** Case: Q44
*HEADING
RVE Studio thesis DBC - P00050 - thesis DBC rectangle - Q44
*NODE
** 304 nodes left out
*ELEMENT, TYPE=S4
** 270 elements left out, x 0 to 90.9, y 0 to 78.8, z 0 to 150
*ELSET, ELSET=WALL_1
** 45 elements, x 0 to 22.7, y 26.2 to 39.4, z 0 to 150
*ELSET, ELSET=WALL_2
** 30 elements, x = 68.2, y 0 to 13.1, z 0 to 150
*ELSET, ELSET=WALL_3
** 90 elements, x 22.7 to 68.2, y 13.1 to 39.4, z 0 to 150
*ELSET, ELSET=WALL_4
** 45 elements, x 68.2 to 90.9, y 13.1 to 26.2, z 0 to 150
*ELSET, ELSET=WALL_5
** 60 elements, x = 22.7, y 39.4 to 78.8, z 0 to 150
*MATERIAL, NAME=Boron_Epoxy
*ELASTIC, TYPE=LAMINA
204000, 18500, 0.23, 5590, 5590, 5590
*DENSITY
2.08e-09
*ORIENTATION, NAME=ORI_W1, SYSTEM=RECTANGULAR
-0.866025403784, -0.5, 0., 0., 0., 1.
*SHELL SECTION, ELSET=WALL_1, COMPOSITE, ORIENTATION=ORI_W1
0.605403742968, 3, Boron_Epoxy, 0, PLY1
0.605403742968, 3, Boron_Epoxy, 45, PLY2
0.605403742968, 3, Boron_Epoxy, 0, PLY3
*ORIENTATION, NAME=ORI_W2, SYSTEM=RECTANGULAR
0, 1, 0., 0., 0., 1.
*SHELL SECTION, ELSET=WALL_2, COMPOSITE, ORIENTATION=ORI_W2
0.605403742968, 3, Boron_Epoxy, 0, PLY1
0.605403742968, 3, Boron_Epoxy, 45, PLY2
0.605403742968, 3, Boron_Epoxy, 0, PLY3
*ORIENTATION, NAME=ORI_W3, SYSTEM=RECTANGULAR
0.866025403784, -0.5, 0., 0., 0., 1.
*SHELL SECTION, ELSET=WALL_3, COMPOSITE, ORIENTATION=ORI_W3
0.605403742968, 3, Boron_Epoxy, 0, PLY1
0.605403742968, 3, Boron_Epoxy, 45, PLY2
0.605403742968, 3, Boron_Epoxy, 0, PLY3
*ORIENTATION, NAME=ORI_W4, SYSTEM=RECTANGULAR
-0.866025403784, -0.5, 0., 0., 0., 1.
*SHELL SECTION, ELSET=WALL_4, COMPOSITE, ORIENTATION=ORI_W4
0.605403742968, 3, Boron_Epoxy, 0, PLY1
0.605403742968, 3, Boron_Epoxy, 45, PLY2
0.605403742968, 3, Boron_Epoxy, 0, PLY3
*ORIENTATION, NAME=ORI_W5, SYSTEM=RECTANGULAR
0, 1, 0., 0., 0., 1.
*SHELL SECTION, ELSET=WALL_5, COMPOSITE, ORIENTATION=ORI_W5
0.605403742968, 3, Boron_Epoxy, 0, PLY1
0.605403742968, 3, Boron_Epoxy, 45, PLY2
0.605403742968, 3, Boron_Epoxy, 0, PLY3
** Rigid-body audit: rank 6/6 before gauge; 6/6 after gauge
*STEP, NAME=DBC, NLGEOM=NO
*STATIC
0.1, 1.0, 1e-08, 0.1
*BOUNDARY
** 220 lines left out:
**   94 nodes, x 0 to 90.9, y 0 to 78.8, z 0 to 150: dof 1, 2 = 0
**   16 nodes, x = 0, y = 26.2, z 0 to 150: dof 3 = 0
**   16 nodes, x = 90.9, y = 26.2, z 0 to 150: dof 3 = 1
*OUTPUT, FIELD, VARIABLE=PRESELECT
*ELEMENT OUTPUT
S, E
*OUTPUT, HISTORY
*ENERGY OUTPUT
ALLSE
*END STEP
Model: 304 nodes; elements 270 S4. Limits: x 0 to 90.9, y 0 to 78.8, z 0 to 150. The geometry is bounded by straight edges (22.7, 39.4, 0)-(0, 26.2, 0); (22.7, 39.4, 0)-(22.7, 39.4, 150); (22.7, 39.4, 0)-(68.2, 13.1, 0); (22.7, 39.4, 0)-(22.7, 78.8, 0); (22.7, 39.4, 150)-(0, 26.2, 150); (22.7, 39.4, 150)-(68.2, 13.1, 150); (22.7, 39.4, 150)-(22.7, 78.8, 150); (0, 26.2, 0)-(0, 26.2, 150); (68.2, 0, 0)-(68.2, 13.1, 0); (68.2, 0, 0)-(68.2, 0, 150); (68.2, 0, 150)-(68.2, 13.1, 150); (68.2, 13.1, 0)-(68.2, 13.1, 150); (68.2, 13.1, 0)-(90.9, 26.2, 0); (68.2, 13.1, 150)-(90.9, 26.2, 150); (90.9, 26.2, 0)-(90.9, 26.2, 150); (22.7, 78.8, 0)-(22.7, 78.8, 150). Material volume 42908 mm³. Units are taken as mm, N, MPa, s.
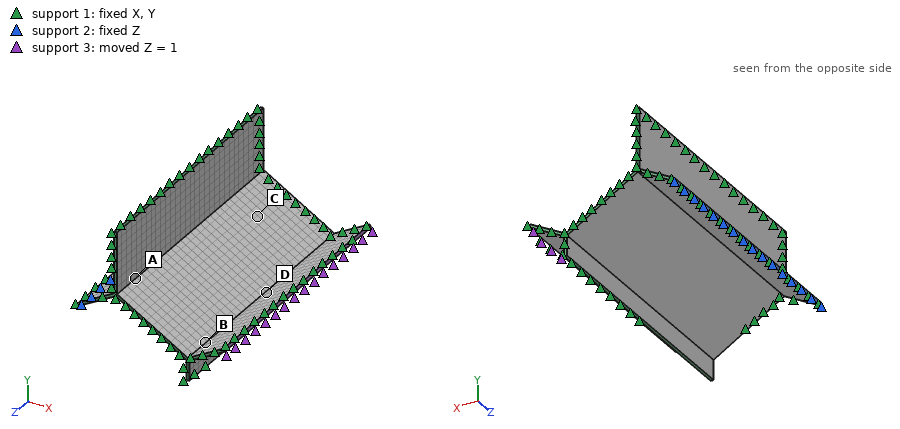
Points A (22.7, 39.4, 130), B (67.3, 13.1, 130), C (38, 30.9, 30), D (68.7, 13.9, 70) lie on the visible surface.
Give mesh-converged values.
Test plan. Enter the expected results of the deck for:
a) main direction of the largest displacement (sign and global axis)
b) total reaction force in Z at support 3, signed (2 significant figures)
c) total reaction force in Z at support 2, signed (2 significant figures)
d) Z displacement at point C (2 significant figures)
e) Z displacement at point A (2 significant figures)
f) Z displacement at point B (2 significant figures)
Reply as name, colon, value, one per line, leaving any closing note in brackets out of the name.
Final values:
main direction of the largest displacement: +Z
total reaction force in Z at support 3, signed: 50000 N
total reaction force in Z at support 2, signed: -50000 N
Z displacement at point C: 0.45 mm
Z displacement at point A: 0.22 mm
Z displacement at point B: 0.73 mm
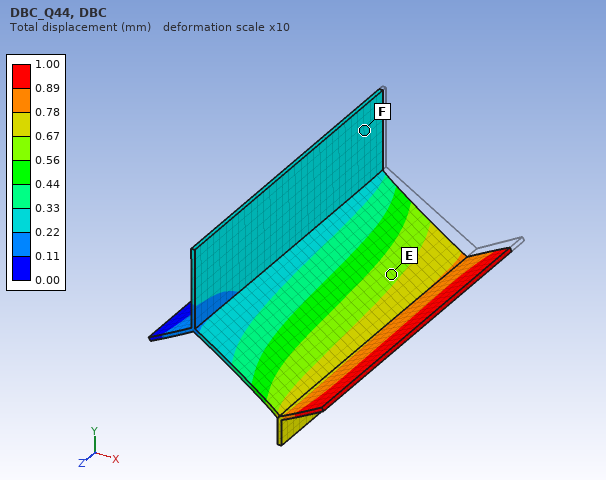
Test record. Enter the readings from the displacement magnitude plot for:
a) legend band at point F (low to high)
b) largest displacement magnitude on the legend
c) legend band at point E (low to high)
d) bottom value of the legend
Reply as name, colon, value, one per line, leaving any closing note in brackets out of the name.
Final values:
legend band at point F: 0.22 to 0.33 mm
largest displacement magnitude on the legend: 1.00 mm
legend band at point E: 0.56 to 0.67 mm
bottom value of the legend: 0.00 mm
